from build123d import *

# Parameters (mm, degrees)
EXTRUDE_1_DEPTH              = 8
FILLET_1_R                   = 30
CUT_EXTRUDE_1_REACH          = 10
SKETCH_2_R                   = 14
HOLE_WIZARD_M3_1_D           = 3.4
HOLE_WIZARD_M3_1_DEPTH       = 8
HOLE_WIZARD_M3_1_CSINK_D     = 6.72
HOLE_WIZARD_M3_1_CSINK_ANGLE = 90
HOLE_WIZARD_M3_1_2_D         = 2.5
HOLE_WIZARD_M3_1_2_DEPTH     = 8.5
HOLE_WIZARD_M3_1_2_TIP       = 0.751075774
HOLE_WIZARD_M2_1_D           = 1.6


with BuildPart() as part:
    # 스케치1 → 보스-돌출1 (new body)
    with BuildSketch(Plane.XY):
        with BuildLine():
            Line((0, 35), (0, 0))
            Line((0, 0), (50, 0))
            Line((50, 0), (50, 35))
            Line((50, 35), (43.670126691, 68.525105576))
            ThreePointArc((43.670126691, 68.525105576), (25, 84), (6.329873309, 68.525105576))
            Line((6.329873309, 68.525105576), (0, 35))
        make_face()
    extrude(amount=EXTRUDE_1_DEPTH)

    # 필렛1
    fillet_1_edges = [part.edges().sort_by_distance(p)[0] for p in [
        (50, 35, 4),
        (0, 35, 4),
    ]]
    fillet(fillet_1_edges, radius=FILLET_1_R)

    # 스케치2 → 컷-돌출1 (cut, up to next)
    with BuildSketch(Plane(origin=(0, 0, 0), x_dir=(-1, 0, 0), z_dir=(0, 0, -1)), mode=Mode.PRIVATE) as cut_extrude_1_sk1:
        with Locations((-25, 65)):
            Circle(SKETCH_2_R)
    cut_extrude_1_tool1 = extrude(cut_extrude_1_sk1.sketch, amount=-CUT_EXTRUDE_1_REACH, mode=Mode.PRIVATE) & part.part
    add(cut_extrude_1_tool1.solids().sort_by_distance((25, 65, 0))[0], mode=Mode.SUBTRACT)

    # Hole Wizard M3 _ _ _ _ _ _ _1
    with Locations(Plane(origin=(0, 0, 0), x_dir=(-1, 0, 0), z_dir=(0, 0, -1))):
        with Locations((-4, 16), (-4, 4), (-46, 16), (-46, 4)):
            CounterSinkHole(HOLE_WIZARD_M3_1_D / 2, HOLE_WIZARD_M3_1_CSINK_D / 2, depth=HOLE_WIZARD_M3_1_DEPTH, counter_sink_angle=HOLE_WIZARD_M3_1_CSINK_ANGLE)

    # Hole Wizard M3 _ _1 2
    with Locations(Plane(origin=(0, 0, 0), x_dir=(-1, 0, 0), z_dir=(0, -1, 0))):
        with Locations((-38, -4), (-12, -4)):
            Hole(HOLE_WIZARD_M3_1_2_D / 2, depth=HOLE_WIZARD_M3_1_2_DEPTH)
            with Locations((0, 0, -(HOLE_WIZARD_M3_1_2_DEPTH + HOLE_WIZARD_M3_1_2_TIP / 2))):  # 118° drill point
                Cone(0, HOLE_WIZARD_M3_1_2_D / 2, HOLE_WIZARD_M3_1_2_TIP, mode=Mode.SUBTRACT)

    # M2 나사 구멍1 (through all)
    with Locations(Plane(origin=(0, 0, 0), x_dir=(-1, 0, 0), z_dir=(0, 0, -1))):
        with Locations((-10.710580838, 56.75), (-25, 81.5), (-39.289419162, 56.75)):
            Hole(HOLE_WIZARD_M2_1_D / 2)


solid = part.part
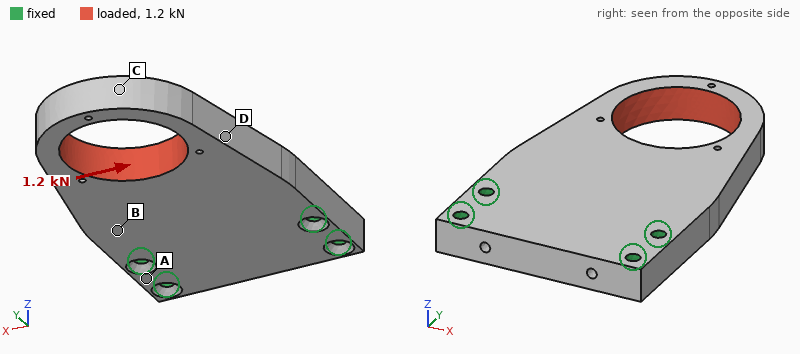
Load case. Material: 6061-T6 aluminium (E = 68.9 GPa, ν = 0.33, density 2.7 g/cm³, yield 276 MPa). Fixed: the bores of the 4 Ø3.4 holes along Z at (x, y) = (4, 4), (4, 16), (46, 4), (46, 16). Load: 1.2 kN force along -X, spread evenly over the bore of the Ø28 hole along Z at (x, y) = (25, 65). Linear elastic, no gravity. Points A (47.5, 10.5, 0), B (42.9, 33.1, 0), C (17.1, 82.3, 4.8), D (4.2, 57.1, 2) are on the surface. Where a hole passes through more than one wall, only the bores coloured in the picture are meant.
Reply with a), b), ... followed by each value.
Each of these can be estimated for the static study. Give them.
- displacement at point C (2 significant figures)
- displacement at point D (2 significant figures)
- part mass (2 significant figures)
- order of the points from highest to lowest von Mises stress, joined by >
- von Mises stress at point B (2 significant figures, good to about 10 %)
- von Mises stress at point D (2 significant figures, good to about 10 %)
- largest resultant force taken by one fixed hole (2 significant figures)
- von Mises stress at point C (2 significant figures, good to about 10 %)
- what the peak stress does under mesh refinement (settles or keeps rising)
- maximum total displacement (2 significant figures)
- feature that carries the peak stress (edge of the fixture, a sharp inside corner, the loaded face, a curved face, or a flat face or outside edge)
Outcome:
a) 56 µm
b) 19 µm
c) 64 g
d) D > C > B > A
e) 8.9 MPa
f) 36 MPa
g) 1.3 kN
h) 21 MPa
i) keeps rising
j) 58 µm
k) edge of the fixture
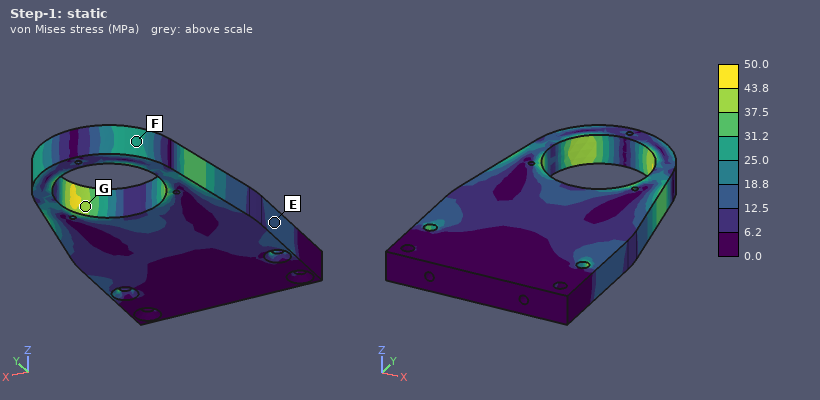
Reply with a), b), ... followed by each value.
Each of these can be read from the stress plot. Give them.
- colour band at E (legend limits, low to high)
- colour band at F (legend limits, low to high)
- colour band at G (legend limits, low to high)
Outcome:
a) 12.5 to 18.8 MPa
b) 25.0 to 31.2 MPa
c) 37.5 to 43.8 MPa
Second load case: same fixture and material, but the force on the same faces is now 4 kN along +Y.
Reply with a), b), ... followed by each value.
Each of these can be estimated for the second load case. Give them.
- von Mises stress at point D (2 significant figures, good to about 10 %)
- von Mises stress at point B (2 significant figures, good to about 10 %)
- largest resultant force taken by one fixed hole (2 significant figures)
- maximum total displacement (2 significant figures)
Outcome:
a) 30 MPa
b) 13 MPa
c) 1.6 kN
d) 37 µm
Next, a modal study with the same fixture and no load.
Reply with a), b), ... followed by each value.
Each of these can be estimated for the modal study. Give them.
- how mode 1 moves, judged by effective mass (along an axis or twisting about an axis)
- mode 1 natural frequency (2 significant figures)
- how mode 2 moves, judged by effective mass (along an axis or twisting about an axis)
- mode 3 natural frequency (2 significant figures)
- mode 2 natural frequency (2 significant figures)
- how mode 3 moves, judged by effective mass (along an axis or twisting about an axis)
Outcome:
a) along Z
b) 2000 Hz
c) twisting about Y
d) 6800 Hz
e) 5600 Hz
f) along Z
